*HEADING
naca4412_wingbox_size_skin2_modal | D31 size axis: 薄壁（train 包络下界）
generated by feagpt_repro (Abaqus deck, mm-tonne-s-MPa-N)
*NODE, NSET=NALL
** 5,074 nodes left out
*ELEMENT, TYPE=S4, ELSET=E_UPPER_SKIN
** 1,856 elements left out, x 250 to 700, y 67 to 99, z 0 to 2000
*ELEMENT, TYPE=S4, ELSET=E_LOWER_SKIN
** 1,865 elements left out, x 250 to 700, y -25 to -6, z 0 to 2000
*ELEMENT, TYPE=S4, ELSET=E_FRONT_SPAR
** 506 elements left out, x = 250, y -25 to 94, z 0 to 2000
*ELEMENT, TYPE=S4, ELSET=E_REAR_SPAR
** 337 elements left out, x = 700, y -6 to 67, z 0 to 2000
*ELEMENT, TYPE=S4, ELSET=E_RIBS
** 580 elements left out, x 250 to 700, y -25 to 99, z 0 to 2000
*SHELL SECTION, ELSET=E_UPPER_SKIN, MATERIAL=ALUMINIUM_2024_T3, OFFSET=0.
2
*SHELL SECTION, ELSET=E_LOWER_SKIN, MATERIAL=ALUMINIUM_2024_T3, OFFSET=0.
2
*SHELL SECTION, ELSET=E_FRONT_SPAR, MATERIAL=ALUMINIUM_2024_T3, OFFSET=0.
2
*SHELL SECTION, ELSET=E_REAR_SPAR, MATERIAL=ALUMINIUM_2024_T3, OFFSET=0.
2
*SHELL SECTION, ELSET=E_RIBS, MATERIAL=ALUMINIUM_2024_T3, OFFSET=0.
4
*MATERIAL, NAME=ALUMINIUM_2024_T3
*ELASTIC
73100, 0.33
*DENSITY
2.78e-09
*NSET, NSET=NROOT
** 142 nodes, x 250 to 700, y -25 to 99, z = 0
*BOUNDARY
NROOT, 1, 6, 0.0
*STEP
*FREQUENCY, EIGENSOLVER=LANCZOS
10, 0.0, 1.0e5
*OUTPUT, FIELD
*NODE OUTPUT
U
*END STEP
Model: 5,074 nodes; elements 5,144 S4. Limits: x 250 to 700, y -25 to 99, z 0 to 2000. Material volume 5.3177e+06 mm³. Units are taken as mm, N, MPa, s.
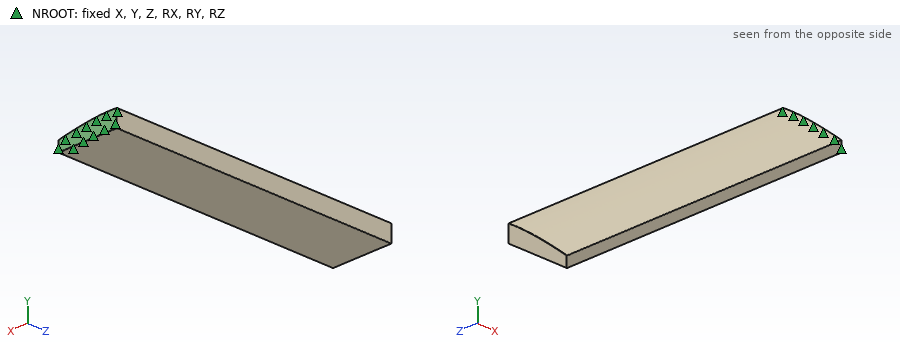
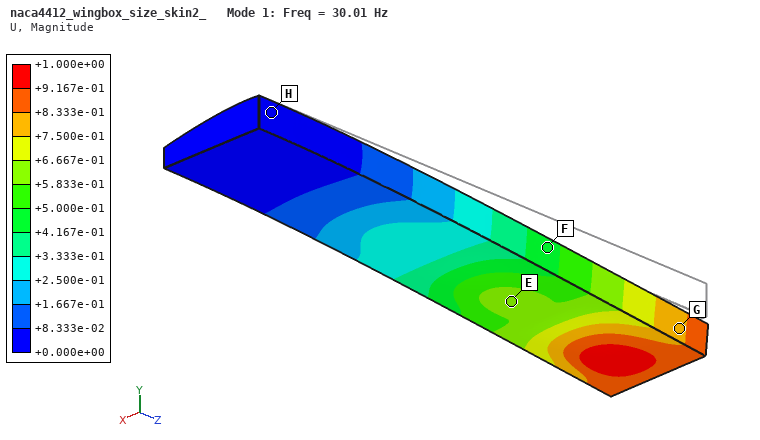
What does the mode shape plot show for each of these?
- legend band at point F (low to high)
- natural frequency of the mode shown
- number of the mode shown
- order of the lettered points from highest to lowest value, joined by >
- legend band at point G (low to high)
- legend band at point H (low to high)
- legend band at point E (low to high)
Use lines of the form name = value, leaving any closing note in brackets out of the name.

legend band at point F = +4.167e-01 to +5.000e-01
natural frequency of the mode shown = 30.01 Hz
number of the mode shown = 1
order of the lettered points from highest to lowest value, joined by > = G > E > F > H
legend band at point G = +7.500e-01 to +8.333e-01
legend band at point H = +0.000e+00 to +8.333e-02
legend band at point E = +5.833e-01 to +6.667e-01
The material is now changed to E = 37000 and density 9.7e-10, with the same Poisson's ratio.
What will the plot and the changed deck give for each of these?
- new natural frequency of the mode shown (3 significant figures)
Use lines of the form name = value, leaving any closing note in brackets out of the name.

new natural frequency of the mode shown = 36.1 Hz
